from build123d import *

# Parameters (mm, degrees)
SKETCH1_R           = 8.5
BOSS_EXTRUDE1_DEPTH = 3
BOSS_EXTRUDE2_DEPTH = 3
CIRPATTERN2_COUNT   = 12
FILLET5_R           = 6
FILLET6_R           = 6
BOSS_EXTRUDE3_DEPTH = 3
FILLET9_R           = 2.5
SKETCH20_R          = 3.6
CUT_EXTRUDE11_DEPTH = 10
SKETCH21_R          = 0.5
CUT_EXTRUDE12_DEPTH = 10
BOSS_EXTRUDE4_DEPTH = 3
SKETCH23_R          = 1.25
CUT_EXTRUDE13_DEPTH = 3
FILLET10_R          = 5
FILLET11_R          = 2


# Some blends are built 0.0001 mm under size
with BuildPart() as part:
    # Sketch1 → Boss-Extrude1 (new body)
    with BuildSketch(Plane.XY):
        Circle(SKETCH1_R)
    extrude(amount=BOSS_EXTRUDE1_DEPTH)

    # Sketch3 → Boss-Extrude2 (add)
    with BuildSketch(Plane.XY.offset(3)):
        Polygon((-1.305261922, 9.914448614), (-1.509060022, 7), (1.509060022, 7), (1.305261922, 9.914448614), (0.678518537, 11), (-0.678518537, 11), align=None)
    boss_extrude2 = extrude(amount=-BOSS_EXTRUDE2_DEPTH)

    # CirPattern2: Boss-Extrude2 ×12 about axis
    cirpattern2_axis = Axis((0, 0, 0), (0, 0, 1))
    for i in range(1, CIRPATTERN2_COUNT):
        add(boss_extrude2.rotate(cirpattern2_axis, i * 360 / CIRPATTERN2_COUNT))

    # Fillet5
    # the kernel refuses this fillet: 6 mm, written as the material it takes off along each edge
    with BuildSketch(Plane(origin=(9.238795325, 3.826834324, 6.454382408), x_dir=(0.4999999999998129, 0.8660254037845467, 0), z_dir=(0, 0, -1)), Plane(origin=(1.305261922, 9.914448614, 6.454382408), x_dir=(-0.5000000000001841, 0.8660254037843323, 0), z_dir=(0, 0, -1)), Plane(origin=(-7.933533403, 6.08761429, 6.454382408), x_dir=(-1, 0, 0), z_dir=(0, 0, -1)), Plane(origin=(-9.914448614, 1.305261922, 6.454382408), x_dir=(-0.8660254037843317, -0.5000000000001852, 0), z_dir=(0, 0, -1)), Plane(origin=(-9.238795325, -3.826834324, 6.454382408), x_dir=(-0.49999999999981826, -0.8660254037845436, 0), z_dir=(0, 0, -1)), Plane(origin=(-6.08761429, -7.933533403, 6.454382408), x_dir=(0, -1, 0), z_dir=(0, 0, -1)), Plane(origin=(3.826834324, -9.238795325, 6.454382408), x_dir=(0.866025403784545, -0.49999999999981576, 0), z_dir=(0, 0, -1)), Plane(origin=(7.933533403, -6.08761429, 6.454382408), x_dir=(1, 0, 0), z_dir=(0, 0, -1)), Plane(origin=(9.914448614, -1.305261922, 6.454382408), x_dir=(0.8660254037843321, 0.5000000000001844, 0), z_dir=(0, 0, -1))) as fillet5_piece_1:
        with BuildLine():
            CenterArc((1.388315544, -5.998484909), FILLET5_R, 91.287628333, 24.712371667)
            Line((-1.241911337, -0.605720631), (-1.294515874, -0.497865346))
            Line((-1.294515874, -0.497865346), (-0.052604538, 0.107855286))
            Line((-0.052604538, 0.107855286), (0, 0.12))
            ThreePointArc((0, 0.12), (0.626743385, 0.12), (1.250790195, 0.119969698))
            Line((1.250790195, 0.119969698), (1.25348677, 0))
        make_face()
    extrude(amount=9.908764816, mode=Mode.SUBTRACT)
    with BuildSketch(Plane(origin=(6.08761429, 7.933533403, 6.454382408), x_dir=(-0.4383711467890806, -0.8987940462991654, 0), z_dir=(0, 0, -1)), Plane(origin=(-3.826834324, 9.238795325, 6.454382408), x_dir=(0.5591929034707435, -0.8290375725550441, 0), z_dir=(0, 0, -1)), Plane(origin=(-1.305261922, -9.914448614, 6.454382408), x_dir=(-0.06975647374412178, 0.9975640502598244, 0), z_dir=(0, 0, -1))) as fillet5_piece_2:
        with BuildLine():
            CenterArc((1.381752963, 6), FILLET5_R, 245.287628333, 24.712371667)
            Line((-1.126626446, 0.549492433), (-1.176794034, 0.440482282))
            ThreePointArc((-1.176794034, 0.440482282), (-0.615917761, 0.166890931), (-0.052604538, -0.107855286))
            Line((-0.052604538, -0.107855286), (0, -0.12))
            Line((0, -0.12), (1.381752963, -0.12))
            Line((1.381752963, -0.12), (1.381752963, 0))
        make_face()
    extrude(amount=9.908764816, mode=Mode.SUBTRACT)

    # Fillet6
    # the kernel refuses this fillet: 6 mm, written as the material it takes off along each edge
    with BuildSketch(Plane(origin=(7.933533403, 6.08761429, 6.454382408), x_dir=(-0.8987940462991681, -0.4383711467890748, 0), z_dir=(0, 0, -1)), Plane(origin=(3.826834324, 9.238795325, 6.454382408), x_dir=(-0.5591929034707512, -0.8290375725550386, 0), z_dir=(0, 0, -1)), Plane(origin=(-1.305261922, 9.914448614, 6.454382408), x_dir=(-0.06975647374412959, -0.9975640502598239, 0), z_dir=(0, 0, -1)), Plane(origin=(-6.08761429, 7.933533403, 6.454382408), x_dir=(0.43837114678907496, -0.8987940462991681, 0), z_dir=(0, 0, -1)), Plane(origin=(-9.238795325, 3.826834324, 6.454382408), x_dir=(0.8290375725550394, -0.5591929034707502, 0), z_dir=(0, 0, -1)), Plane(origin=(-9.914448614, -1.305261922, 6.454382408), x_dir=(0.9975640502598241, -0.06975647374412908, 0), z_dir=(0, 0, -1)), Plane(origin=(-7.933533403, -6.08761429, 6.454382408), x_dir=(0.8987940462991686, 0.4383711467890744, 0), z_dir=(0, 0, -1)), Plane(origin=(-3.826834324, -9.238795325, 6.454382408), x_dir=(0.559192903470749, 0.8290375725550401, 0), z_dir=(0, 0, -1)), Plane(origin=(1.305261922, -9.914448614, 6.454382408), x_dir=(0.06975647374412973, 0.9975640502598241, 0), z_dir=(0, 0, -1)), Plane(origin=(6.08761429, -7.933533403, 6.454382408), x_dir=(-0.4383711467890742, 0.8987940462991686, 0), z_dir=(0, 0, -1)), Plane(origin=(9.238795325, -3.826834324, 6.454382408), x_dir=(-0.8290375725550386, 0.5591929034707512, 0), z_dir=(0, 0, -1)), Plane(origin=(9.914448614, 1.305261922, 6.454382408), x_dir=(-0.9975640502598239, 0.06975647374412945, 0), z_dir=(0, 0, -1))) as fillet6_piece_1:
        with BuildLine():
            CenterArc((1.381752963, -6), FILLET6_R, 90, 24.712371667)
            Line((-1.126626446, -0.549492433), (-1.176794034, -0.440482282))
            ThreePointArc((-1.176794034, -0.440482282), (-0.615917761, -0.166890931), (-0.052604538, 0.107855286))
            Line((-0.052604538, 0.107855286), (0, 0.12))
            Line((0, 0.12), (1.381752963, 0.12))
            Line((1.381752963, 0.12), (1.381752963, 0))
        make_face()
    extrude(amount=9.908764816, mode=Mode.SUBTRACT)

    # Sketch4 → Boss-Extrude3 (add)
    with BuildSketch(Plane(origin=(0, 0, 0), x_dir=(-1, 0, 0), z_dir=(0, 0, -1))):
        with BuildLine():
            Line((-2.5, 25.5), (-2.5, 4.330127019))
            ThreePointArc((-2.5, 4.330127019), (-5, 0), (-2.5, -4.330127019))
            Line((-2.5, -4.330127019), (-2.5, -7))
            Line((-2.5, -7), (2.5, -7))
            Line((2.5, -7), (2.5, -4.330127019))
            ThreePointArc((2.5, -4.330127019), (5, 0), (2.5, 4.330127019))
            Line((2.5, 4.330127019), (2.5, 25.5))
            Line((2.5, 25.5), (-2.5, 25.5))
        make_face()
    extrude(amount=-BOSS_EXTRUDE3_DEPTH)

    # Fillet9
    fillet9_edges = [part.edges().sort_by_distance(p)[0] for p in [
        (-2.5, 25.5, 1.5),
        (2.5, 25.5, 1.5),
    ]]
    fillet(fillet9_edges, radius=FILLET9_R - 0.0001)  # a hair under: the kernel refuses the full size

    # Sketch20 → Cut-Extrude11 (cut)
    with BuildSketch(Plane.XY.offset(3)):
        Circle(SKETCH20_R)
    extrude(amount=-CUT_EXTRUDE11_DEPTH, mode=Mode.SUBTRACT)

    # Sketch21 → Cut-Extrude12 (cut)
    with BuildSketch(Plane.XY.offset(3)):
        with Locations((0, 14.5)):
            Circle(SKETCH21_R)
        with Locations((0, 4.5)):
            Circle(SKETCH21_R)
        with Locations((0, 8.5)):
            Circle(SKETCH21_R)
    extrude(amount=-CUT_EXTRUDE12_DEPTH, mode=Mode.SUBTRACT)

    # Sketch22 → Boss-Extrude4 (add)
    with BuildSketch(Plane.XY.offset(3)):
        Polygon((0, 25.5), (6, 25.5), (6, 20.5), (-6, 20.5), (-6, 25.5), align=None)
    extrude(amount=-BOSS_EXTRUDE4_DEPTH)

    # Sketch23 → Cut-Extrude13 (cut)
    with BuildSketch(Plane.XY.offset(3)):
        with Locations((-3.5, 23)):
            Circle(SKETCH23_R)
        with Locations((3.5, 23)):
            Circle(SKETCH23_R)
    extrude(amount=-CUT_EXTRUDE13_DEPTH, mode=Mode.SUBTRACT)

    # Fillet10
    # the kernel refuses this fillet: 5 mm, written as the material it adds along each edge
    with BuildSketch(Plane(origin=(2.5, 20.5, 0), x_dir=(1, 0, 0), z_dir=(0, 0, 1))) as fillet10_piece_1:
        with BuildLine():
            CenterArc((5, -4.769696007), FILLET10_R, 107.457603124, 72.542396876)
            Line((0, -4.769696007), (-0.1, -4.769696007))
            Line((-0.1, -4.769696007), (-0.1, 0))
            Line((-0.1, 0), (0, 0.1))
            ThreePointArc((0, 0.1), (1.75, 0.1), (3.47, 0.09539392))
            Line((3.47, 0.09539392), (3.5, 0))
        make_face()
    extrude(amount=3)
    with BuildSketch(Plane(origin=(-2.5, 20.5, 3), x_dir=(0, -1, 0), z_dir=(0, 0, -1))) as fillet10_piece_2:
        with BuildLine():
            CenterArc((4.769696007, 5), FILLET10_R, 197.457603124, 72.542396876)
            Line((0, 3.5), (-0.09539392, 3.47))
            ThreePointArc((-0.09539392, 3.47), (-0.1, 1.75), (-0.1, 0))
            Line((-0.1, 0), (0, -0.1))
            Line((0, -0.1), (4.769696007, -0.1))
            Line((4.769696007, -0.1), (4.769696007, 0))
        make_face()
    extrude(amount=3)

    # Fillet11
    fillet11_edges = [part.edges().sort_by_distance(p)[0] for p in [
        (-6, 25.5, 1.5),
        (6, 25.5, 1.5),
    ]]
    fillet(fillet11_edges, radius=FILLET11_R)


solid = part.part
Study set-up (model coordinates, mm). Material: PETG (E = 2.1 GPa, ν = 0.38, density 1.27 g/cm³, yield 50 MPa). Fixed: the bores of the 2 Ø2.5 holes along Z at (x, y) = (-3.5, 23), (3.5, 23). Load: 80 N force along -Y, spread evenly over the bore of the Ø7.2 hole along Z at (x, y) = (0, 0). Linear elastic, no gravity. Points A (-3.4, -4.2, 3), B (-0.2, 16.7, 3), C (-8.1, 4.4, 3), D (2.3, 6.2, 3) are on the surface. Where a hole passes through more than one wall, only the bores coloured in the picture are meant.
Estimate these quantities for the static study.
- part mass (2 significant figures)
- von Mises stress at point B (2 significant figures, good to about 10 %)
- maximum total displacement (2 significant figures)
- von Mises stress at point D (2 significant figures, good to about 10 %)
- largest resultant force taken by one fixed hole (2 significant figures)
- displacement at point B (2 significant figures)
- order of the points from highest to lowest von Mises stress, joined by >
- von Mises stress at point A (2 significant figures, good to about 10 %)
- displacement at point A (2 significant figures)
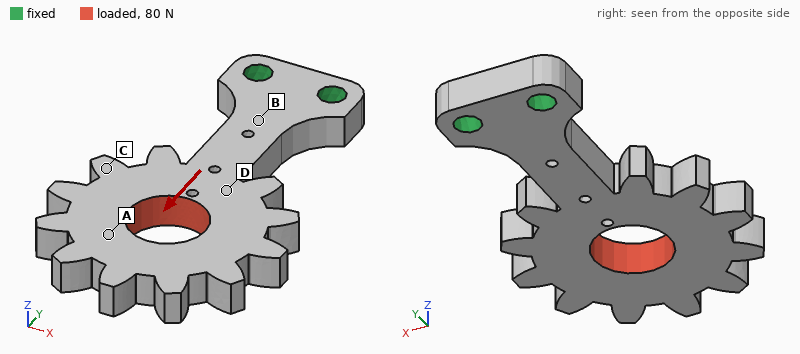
1.4 g
3.7 MPa
68 µm
5.1 MPa
43 N
11 µm
D > B > A > C
1.8 MPa
63 µm
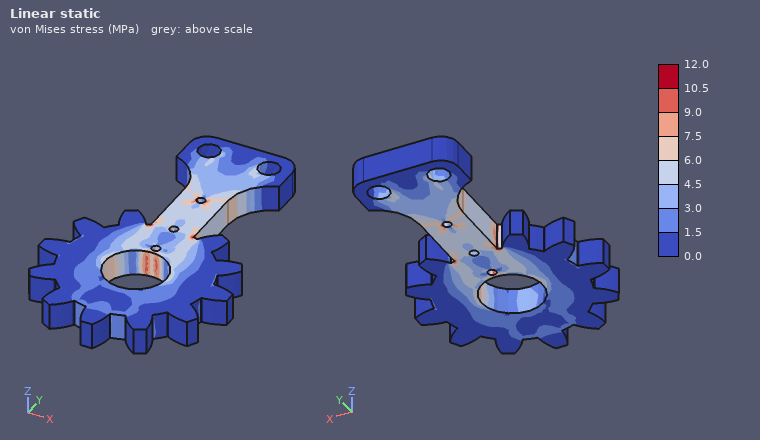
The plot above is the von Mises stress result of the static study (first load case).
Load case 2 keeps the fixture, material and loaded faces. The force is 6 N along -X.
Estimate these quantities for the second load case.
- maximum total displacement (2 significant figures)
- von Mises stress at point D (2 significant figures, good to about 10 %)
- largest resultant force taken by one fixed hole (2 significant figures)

0.39 mm
1.00 MPa
18 N
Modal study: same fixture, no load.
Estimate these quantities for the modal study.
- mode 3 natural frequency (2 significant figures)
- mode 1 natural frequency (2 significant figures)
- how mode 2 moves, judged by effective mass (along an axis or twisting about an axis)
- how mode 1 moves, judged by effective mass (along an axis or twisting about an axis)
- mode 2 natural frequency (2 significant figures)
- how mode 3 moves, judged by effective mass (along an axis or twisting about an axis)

1100 Hz
410 Hz
along X
along Z
740 Hz
twisting about Y
